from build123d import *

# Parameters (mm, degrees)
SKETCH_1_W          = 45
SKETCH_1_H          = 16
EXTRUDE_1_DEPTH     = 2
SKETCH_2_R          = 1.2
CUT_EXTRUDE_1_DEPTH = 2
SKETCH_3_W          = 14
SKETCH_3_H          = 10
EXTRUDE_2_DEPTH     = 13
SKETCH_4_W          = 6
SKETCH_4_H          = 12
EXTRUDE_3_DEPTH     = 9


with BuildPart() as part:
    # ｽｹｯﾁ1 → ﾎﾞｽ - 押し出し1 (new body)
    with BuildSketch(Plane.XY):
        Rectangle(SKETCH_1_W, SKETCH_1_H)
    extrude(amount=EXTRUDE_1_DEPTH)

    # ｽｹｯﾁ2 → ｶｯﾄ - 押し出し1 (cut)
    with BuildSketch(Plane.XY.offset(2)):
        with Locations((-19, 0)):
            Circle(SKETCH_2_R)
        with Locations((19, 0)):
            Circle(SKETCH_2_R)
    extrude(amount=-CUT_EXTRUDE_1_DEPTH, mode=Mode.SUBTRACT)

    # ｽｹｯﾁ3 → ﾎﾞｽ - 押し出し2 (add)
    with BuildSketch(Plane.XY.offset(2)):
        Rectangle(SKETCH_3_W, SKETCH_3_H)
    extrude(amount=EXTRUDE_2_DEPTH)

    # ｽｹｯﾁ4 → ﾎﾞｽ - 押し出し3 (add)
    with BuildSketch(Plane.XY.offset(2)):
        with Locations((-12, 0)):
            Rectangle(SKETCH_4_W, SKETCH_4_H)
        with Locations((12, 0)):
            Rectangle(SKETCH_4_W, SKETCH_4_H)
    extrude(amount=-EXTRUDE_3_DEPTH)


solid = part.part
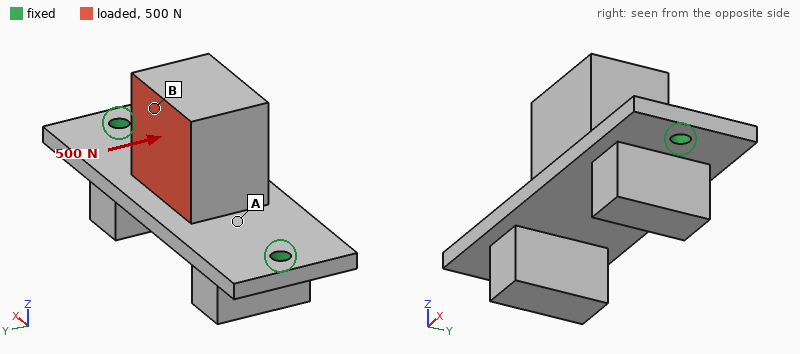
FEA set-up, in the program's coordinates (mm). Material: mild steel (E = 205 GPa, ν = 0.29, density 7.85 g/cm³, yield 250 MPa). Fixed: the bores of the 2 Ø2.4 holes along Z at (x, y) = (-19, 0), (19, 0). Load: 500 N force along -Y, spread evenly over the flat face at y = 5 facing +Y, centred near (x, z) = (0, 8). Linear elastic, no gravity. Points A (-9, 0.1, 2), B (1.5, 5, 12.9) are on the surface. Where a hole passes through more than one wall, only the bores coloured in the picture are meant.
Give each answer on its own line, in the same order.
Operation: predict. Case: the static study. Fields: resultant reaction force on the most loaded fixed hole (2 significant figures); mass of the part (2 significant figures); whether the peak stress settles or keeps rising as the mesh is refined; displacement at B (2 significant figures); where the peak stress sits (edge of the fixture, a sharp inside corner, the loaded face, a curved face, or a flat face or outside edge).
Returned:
250 N
33 g
keeps rising
50 µm
edge of the fixture
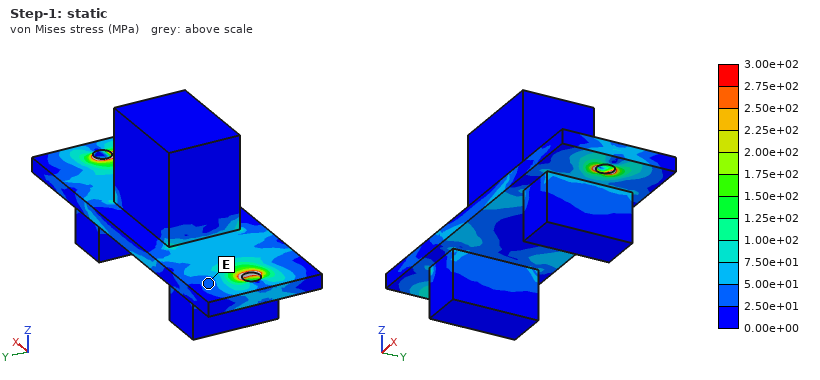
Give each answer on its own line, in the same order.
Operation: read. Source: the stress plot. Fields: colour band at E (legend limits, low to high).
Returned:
2.50e+01 to 5.00e+01 MPa
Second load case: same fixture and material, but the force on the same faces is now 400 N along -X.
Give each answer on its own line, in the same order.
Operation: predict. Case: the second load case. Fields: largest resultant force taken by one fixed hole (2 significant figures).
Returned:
230 N
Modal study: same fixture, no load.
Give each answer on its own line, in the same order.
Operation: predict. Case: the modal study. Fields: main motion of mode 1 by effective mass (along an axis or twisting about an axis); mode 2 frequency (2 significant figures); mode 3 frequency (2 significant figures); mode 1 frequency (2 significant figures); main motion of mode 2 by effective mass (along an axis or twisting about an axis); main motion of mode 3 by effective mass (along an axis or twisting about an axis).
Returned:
along Y
4500 Hz
7300 Hz
4200 Hz
along Z
along X
